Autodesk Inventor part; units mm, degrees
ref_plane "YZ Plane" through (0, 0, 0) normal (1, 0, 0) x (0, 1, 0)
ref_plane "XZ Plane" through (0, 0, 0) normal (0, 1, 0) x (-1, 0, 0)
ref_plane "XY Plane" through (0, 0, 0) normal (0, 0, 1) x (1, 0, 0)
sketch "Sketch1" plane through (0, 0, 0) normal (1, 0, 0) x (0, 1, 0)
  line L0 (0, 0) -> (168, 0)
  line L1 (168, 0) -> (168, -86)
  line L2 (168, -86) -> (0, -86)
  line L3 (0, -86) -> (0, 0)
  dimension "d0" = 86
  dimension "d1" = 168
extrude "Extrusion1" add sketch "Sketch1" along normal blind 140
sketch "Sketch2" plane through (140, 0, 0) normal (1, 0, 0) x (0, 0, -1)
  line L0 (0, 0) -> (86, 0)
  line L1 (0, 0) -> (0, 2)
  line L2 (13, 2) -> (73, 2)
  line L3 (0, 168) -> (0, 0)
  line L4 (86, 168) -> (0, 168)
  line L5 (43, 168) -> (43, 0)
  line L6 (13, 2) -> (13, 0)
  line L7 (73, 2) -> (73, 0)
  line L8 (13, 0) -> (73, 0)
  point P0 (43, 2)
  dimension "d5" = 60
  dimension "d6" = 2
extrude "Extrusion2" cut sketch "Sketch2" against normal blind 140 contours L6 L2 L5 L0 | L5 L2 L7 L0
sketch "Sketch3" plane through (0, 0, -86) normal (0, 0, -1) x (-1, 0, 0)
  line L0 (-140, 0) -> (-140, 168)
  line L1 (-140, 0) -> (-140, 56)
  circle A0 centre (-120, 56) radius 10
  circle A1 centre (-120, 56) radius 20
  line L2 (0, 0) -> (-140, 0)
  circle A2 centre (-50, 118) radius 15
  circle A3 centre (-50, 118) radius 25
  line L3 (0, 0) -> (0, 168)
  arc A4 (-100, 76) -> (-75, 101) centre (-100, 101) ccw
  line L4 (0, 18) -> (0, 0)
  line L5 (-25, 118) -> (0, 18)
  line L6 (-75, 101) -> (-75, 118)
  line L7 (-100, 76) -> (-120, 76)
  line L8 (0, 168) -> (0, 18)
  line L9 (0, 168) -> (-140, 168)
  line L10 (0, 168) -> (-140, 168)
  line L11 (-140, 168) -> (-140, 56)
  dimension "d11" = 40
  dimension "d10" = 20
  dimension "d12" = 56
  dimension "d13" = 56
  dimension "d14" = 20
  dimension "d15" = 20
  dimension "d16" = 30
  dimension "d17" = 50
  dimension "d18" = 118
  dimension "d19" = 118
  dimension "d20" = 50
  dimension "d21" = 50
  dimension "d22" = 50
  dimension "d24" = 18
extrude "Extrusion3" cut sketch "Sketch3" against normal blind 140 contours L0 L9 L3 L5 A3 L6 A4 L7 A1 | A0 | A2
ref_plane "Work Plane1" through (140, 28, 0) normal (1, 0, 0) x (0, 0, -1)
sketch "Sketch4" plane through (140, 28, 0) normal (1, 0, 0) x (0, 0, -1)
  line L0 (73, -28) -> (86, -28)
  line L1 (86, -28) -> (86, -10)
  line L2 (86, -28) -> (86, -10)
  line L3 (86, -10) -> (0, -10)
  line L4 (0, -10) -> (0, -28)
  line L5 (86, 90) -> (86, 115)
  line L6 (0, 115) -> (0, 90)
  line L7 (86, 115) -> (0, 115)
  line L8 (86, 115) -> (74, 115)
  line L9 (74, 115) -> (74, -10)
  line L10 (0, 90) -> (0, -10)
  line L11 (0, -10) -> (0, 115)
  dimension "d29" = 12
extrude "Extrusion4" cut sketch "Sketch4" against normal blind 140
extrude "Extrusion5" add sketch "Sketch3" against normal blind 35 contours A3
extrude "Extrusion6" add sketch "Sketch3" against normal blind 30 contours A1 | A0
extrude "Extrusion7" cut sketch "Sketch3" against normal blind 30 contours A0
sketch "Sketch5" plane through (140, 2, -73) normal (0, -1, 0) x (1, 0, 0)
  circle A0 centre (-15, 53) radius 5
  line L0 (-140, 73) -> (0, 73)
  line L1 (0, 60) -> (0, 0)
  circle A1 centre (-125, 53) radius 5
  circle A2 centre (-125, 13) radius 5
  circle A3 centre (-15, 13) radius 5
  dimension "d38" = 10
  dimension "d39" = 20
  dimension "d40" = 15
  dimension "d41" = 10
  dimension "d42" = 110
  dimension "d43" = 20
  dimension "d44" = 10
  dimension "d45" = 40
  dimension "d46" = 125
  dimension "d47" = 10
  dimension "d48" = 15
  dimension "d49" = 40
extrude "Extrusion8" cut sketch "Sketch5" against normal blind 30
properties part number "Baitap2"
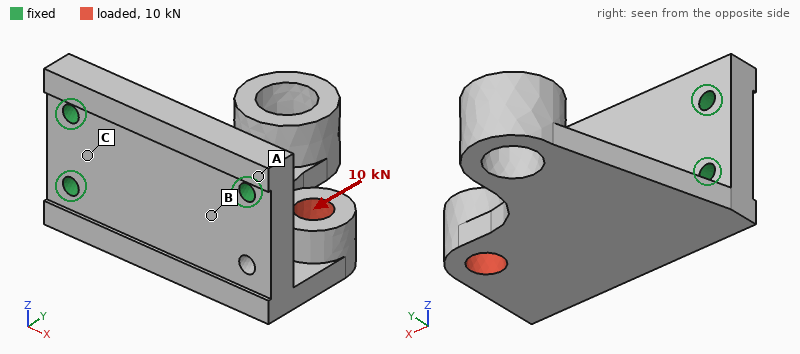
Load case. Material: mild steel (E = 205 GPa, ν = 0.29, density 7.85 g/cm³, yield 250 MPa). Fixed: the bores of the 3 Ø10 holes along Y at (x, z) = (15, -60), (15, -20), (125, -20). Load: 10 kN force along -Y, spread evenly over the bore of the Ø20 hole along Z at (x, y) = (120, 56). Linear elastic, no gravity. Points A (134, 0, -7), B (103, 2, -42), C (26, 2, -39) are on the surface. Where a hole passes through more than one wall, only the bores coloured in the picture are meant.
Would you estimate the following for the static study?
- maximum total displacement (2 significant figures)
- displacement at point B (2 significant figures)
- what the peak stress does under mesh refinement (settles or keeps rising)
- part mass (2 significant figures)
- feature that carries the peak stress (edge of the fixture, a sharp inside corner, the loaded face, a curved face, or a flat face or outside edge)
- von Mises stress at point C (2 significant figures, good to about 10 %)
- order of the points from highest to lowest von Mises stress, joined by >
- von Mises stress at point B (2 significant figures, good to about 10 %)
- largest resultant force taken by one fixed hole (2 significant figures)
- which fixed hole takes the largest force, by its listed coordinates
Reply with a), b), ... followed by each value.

a) 0.15 mm
b) 0.026 mm
c) keeps rising
d) 2.8 kg
e) edge of the fixture
f) 30 MPa
g) B > C > A
h) 55 MPa
i) 8.2 kN
j) (125, -20)
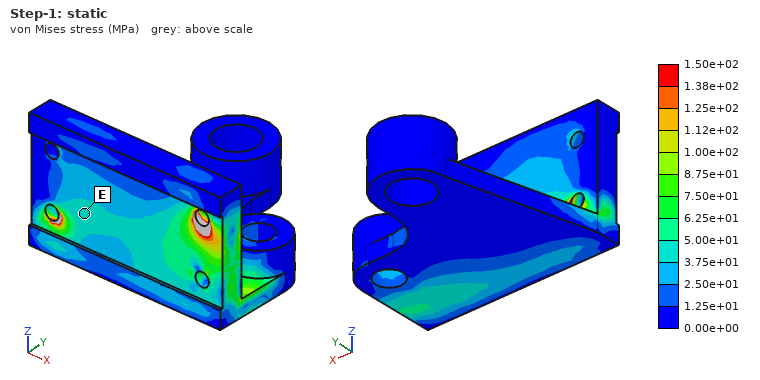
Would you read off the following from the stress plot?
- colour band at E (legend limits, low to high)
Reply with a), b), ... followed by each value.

a) 3.75e+01 to 5.00e+01 MPa
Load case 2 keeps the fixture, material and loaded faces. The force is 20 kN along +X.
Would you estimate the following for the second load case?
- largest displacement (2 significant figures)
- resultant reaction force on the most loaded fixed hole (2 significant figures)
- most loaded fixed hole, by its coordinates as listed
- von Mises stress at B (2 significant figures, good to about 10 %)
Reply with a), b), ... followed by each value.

a) 0.21 mm
b) 14 kN
c) (15, -60)
d) 53 MPa
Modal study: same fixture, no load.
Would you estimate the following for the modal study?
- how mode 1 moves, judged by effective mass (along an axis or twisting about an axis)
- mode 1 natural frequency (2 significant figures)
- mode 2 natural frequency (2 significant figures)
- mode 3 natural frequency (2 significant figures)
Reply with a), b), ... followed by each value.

a) along Z
b) 590 Hz
c) 1200 Hz
d) 2300 Hz
